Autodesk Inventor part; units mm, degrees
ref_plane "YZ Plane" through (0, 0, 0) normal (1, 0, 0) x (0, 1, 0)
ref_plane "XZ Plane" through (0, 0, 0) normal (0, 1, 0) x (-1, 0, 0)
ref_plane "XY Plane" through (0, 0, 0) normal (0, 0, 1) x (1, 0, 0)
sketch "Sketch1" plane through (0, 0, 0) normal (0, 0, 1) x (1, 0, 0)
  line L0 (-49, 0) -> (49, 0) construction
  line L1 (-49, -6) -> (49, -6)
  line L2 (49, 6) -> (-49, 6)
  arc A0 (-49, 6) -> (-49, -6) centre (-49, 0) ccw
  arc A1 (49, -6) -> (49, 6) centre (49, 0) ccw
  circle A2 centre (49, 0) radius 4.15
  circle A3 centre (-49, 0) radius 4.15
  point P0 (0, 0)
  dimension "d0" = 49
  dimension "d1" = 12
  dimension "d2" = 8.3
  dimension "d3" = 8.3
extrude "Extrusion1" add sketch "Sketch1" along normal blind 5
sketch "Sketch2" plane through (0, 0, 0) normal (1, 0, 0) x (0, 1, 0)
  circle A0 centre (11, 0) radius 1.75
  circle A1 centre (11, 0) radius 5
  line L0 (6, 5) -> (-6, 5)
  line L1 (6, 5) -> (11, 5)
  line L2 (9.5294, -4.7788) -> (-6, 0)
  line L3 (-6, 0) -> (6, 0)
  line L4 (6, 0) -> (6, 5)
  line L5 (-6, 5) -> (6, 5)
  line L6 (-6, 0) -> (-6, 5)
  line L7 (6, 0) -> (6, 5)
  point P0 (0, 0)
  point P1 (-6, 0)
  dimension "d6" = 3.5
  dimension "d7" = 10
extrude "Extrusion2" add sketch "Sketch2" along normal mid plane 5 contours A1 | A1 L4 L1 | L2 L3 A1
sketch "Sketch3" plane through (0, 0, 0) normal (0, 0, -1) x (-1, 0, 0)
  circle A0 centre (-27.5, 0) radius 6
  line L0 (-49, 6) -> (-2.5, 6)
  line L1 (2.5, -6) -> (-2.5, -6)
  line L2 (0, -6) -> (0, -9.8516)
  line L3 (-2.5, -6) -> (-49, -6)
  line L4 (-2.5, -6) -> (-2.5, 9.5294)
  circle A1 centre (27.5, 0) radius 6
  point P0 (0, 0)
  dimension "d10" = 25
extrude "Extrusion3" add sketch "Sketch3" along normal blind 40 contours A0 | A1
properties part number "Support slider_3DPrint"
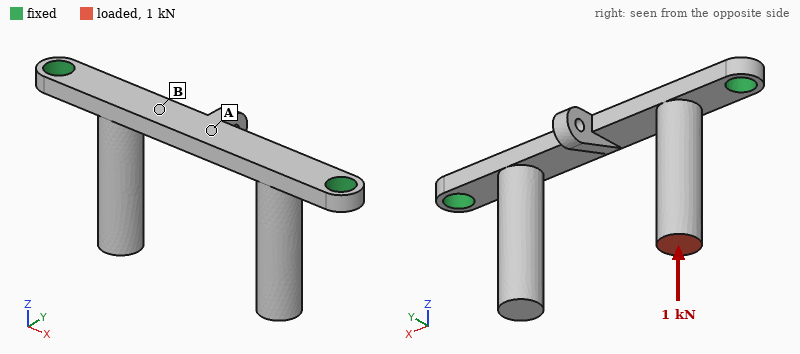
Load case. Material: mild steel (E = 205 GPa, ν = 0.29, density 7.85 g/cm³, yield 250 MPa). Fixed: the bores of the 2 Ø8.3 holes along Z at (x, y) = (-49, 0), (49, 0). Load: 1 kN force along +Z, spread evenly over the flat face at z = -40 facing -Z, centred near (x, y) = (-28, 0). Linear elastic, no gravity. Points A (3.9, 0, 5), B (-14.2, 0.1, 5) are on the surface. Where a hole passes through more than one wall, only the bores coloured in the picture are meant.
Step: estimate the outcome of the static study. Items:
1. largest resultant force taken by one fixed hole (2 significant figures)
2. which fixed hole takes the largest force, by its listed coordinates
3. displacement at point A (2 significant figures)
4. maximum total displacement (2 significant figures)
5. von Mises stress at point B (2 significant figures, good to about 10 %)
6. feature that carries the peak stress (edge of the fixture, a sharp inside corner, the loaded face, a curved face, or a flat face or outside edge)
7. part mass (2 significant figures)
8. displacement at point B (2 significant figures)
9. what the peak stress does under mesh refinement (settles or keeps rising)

880 N
(-49, 0)
0.052 mm
0.11 mm
71 MPa
edge of the fixture
120 g
0.060 mm
keeps rising
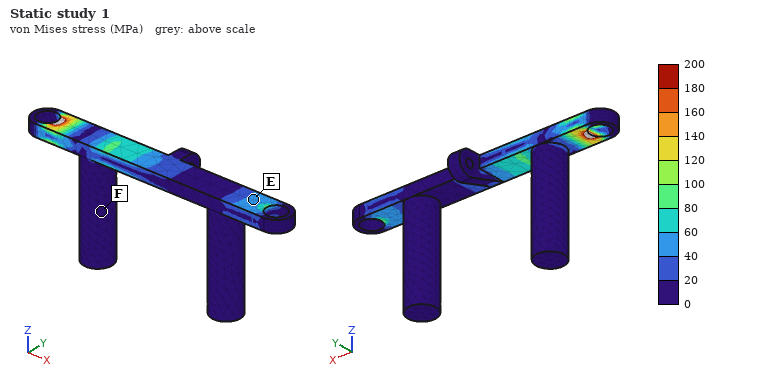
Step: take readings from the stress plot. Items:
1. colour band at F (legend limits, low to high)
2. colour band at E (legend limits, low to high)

0 to 20 MPa
40 to 60 MPa
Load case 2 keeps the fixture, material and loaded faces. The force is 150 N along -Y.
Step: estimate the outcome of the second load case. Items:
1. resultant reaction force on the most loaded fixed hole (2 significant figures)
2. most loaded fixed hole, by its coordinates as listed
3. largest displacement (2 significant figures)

140 N
(-49, 0)
0.12 mm
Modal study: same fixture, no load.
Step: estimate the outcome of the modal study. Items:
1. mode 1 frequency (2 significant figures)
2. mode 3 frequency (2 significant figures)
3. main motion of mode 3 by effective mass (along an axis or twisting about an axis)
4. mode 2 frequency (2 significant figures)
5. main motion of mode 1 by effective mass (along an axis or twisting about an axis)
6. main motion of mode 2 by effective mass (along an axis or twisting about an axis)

1400 Hz
1800 Hz
twisting about Z
1500 Hz
along Z
along Y
